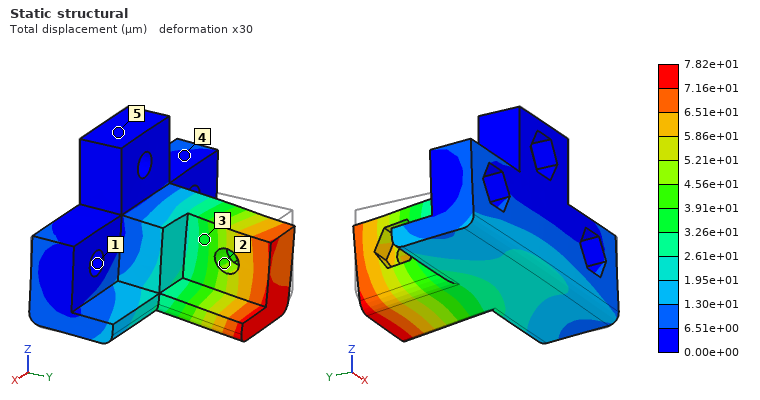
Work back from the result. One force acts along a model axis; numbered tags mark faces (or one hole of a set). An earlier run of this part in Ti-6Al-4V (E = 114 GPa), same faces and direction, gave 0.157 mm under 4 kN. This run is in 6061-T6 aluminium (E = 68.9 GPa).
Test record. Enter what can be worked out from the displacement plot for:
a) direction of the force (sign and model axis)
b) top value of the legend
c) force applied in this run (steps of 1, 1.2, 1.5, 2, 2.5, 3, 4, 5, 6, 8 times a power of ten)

-Z
7.82e+01 µm
1.2 kN
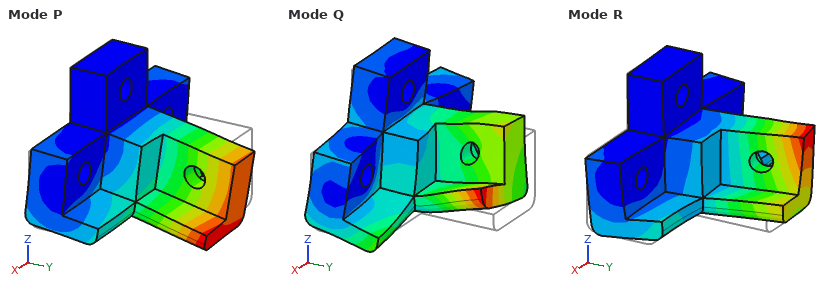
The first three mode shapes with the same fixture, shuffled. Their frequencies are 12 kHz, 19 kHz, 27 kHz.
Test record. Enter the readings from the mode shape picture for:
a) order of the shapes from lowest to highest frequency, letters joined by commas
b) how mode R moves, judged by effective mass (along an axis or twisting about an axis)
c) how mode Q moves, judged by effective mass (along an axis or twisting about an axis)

P, R, Q
along X
along Y
